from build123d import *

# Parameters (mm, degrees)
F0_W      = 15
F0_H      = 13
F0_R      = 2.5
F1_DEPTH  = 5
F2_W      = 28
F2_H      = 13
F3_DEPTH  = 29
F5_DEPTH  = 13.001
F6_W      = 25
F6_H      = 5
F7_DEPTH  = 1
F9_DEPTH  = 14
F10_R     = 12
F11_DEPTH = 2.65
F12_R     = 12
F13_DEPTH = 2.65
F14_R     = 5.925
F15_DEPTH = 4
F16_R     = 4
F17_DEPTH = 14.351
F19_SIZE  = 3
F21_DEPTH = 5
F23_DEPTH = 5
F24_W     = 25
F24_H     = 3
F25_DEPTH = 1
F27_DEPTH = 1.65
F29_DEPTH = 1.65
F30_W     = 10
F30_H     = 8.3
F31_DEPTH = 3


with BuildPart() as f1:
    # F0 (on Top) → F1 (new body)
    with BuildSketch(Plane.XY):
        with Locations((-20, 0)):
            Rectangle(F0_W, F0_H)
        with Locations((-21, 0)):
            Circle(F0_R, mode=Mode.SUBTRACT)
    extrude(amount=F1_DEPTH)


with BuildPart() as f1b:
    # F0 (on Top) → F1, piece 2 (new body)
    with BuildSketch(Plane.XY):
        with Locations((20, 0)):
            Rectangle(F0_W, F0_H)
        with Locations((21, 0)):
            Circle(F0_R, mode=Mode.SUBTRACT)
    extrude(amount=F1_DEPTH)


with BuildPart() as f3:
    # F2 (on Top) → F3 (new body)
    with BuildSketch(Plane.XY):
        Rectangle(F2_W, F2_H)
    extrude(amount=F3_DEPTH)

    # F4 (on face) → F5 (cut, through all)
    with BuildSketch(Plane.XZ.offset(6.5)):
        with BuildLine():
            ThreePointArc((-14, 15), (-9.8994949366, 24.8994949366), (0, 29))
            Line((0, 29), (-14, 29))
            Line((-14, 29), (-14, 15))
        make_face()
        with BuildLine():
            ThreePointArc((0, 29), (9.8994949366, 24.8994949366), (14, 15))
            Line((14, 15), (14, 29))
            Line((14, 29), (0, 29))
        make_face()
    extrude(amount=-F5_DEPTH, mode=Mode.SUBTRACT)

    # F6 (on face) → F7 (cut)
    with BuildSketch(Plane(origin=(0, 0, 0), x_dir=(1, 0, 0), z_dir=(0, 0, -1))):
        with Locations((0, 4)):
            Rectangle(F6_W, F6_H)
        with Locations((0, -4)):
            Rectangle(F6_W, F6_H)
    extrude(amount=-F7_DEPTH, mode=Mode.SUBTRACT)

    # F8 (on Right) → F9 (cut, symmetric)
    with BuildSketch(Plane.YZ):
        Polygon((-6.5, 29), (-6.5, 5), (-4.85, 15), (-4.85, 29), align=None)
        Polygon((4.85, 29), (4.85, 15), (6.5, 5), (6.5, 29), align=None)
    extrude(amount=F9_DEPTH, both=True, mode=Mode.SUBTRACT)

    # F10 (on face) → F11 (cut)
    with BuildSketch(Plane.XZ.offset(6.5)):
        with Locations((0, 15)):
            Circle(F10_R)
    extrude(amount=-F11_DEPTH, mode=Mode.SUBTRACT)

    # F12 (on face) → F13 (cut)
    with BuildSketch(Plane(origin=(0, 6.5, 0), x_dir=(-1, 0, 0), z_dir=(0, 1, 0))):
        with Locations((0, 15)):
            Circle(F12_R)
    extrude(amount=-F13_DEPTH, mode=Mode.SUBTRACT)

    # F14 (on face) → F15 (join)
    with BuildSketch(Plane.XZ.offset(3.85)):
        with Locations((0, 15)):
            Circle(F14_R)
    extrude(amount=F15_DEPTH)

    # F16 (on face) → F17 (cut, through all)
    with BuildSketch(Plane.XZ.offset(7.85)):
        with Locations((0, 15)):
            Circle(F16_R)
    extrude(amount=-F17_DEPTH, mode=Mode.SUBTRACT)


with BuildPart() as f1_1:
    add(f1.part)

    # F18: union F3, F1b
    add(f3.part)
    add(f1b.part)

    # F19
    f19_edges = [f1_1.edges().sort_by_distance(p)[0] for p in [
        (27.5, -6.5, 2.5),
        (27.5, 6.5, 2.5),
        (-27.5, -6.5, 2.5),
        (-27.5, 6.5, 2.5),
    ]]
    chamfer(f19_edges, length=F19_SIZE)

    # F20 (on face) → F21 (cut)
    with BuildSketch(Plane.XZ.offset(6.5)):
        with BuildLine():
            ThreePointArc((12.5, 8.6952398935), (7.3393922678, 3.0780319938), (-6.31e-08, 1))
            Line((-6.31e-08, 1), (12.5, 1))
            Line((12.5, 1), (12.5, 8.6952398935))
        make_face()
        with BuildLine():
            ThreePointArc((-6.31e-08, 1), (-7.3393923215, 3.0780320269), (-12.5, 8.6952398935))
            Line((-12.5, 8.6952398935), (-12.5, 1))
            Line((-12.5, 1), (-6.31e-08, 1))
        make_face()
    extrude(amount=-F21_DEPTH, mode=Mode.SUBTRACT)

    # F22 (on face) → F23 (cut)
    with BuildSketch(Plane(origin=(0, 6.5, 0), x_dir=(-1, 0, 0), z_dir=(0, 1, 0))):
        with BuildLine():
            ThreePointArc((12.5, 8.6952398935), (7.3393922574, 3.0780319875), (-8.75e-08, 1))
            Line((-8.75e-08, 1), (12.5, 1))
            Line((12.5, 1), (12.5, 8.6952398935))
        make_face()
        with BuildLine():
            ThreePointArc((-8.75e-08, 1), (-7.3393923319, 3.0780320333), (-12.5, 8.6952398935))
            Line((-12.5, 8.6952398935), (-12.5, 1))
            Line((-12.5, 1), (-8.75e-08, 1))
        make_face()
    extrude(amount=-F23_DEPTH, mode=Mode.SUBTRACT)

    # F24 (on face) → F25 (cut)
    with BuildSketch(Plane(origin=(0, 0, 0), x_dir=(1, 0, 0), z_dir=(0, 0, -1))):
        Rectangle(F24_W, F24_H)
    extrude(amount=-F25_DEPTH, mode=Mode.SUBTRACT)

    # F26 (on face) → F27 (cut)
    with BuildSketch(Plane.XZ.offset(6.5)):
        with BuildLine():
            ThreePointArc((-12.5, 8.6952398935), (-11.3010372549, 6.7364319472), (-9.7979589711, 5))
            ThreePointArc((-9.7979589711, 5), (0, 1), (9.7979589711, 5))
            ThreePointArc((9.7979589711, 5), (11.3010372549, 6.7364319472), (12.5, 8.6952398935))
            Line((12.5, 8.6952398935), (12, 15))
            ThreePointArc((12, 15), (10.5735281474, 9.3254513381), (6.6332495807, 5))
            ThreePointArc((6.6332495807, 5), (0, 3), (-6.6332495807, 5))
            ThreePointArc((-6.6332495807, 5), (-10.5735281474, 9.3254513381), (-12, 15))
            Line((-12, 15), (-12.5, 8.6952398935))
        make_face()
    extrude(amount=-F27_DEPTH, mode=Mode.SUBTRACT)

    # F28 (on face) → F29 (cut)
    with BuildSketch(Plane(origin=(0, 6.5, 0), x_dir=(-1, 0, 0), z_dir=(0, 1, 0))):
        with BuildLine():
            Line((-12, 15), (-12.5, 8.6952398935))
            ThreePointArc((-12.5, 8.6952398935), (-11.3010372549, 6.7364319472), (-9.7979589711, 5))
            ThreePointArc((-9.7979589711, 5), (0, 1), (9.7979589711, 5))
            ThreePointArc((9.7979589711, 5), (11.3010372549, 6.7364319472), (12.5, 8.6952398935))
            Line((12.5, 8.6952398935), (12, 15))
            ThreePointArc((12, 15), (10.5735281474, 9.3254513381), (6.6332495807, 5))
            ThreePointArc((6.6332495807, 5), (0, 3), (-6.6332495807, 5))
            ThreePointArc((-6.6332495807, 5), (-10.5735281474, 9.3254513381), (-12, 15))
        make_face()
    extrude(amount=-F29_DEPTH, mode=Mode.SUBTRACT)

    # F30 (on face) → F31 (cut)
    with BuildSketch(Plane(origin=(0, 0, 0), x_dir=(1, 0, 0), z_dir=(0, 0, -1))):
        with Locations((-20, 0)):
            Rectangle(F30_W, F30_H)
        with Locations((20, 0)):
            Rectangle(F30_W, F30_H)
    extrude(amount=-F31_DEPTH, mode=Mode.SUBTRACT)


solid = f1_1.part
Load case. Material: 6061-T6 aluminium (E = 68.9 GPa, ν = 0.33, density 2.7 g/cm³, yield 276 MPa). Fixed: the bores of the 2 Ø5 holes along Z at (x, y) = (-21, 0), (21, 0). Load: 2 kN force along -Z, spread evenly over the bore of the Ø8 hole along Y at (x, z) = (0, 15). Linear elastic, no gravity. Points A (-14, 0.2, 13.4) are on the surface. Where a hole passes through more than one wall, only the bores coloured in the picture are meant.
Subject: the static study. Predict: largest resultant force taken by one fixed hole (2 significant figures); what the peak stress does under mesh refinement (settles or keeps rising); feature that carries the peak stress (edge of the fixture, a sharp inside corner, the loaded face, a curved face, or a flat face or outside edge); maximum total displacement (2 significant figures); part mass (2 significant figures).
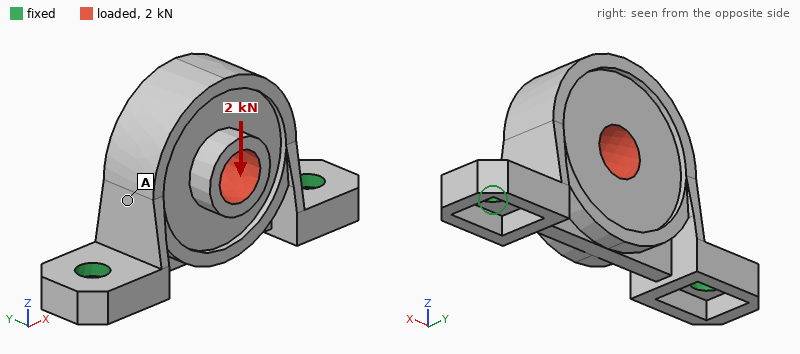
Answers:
1.0 kN
keeps rising
edge of the fixture
0.14 mm
18 g
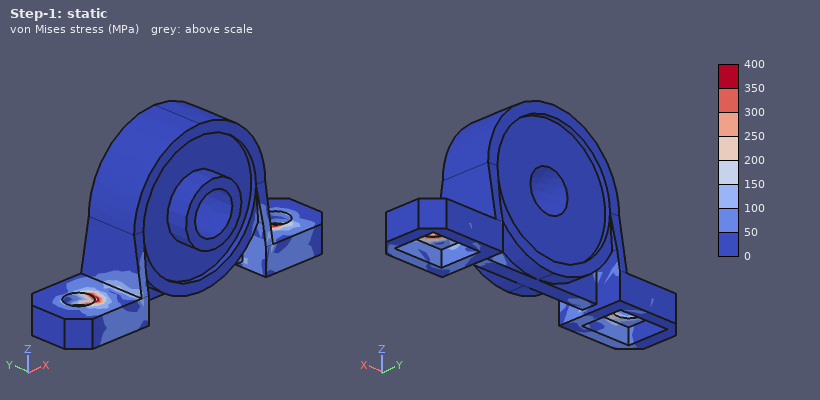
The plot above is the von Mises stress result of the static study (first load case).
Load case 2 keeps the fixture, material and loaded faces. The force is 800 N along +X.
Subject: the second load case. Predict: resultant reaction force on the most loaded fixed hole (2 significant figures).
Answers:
490 N
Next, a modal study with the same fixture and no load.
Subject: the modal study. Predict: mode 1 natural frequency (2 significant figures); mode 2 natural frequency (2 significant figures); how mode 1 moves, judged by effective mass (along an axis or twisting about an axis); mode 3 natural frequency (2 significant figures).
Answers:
2900 Hz
8800 Hz
along Y
9100 Hz
